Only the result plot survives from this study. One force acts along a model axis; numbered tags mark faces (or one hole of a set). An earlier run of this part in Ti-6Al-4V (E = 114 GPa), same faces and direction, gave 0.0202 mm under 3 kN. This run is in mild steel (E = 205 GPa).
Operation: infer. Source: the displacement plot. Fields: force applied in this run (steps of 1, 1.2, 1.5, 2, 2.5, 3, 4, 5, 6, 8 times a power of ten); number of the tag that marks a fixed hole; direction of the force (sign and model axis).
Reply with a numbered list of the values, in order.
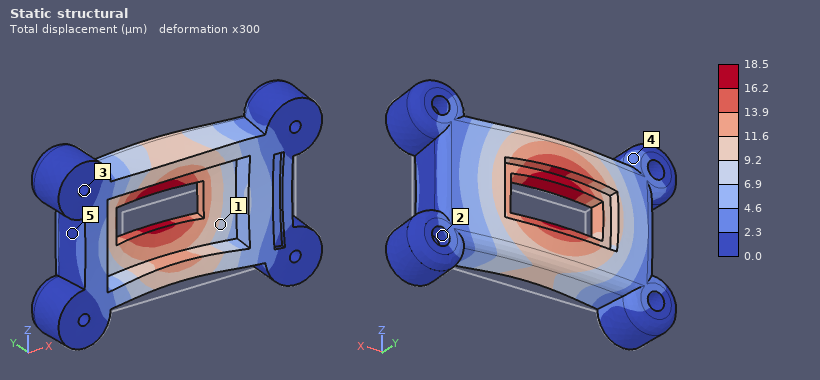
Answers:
1. 5 kN
2. 3
3. +Y
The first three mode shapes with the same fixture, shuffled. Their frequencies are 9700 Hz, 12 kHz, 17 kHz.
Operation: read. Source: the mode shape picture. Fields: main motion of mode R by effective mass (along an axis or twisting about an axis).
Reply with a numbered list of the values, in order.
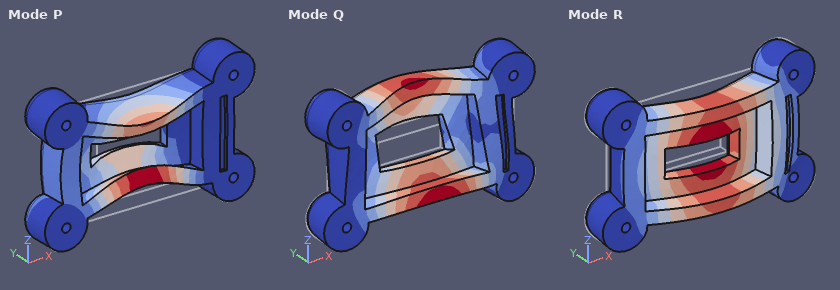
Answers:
1. along Y
